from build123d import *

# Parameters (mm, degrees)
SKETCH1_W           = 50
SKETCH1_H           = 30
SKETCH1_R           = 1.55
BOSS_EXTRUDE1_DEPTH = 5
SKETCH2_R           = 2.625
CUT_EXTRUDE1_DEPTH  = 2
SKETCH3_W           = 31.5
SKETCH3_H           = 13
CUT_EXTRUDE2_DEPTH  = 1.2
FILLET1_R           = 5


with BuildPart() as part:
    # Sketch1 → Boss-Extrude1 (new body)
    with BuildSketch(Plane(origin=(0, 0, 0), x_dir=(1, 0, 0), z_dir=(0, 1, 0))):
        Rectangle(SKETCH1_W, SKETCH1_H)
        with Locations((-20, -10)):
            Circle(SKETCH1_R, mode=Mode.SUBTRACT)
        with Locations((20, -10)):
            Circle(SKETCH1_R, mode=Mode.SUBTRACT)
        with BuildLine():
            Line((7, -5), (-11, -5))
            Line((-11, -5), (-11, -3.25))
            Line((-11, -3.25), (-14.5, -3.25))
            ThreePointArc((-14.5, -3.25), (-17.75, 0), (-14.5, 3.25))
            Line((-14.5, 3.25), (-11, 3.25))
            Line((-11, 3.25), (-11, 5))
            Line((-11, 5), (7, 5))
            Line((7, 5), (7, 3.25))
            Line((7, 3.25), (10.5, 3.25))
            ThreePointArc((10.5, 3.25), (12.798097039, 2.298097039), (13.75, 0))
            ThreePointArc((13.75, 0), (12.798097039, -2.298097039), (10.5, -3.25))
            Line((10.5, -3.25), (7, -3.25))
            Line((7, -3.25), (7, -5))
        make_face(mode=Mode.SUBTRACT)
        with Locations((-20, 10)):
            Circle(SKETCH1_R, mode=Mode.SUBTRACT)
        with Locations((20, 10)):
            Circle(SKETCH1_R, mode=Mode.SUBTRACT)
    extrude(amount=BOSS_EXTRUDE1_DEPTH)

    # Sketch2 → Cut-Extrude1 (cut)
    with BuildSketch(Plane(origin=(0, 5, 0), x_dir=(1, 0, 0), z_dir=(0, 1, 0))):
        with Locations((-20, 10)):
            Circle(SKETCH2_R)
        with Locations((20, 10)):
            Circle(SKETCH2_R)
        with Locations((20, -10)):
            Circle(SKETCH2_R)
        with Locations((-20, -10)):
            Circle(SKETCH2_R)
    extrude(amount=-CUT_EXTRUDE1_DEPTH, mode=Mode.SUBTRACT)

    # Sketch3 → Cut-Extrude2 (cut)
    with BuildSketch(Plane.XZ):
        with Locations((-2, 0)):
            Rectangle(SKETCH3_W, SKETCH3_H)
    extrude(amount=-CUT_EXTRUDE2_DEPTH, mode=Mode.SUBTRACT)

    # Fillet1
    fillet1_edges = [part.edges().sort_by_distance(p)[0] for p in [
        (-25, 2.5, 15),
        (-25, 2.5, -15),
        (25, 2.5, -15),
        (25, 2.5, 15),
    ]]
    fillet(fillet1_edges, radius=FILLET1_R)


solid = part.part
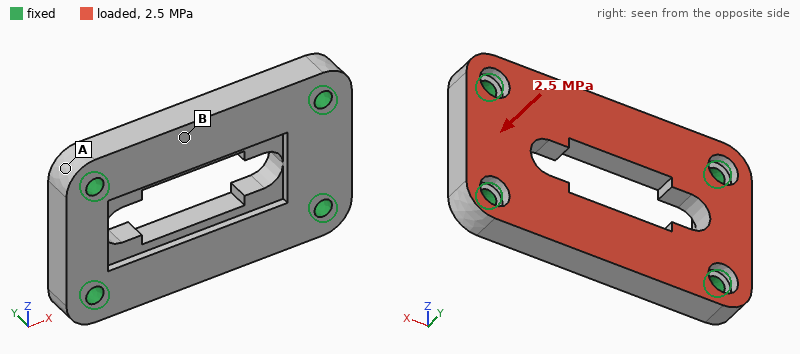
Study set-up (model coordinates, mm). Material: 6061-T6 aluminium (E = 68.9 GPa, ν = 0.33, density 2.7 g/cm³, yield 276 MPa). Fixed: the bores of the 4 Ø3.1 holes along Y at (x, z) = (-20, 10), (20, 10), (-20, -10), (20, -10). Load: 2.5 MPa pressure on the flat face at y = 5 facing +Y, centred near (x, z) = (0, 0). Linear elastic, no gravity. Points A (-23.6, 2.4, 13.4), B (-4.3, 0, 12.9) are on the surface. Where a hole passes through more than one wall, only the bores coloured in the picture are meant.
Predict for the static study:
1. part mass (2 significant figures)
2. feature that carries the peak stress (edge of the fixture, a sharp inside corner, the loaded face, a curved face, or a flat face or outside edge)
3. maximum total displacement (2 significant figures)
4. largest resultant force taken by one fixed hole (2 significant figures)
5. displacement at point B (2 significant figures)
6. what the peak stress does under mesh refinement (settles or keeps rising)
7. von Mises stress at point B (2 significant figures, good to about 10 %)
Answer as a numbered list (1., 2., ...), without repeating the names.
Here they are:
1. 15 g
2. edge of the fixture
3. 41 µm
4. 810 N
5. 34 µm
6. keeps rising
7. 38 MPa
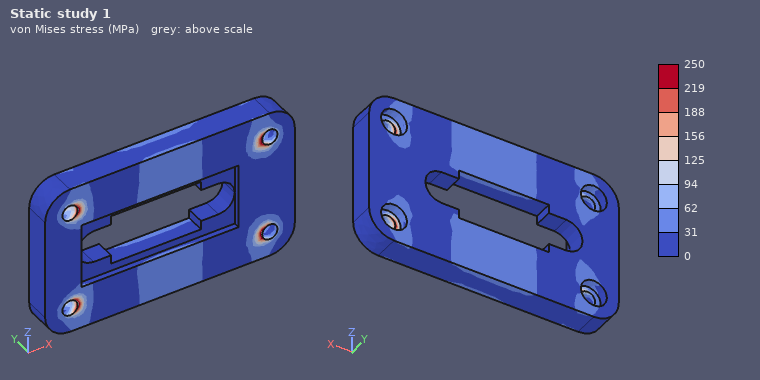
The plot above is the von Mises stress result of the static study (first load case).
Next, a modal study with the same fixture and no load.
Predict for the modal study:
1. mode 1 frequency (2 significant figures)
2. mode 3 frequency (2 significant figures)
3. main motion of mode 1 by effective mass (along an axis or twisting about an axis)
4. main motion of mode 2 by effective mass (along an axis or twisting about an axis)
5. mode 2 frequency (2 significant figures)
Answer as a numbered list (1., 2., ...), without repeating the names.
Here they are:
1. 13 kHz
2. 23 kHz
3. along Y
4. twisting about X
5. 14 kHz
